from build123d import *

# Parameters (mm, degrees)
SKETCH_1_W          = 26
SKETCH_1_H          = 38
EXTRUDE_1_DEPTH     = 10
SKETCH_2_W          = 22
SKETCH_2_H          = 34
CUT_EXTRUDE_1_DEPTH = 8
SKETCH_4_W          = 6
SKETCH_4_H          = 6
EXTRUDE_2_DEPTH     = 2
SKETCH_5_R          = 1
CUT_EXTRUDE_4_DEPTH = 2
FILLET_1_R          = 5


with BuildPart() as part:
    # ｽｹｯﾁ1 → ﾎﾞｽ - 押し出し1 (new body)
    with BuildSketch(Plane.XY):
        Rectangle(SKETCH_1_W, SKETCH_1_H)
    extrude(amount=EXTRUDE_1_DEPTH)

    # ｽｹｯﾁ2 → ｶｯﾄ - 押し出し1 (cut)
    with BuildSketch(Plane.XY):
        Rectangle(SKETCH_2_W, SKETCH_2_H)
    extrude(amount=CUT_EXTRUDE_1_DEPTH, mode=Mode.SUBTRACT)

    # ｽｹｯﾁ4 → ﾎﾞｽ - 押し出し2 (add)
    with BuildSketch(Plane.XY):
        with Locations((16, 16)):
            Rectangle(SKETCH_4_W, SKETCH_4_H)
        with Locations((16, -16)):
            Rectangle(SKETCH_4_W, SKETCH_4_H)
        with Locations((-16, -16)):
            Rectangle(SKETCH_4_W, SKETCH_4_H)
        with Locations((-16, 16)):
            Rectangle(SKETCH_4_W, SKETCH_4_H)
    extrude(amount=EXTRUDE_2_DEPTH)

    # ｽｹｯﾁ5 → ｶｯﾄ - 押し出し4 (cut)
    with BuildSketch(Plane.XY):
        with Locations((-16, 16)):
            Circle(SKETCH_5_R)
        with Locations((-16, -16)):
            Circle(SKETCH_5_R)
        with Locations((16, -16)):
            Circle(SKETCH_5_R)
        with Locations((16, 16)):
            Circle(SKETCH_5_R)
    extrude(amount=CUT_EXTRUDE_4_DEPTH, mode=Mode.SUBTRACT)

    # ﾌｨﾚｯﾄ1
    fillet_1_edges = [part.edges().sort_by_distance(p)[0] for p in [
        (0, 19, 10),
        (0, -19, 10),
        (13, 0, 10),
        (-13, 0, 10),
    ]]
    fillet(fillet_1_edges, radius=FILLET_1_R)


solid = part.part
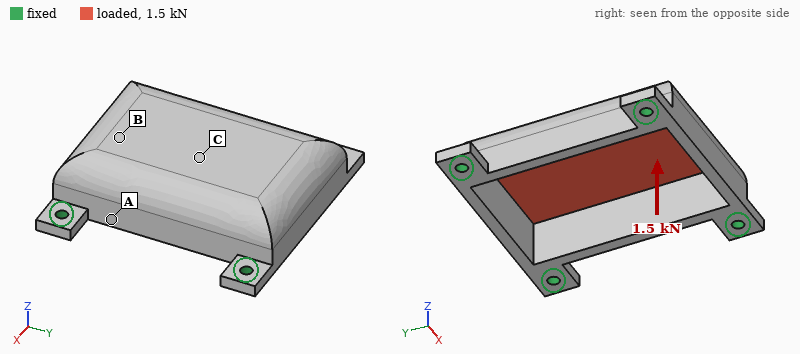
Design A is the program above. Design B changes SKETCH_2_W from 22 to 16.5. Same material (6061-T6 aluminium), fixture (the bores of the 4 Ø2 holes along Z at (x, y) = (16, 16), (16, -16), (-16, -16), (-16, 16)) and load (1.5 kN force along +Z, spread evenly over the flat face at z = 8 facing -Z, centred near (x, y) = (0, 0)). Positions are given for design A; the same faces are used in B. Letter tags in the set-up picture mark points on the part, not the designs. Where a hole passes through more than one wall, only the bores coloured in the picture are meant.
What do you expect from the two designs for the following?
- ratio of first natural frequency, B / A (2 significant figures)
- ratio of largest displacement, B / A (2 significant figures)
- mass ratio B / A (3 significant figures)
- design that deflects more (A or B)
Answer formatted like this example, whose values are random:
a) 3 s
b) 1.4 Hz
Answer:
a) 1.1
b) 0.48
c) 1.42
d) A
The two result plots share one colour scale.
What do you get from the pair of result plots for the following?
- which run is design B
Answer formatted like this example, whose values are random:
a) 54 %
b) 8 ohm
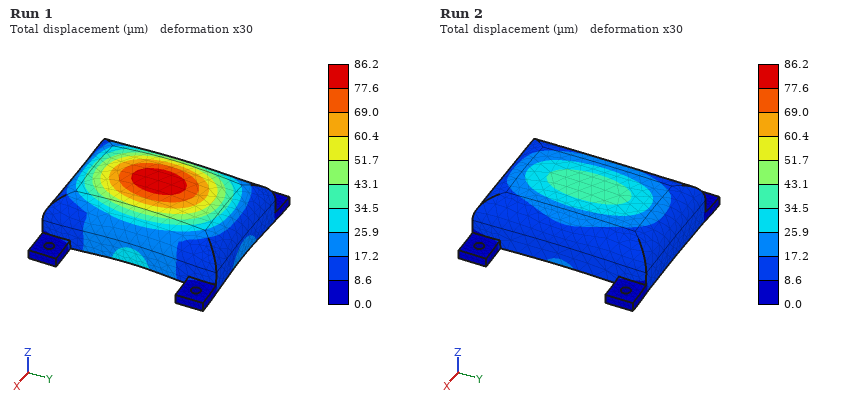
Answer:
a) Run 2
